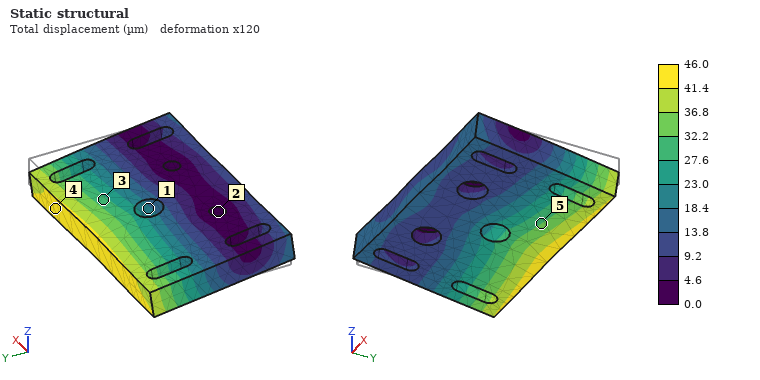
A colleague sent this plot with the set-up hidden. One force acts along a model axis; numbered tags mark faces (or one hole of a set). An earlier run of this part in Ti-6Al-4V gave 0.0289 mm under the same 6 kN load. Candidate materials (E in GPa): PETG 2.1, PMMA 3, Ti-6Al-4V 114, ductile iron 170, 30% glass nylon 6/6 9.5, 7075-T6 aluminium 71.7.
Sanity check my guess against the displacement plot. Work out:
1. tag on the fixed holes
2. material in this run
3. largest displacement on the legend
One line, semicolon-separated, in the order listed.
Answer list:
2; 7075-T6 aluminium; 46.0 µm
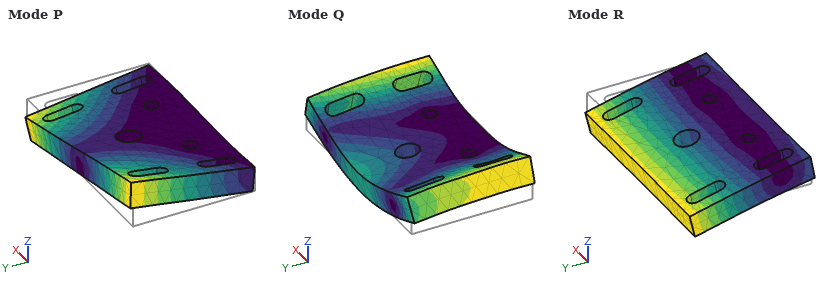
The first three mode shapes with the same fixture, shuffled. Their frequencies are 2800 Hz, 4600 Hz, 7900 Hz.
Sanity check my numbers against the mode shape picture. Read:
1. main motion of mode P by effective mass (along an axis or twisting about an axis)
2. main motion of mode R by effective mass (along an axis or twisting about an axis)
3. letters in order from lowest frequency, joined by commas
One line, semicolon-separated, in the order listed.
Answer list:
twisting about Y; along Z; R, P, Q
